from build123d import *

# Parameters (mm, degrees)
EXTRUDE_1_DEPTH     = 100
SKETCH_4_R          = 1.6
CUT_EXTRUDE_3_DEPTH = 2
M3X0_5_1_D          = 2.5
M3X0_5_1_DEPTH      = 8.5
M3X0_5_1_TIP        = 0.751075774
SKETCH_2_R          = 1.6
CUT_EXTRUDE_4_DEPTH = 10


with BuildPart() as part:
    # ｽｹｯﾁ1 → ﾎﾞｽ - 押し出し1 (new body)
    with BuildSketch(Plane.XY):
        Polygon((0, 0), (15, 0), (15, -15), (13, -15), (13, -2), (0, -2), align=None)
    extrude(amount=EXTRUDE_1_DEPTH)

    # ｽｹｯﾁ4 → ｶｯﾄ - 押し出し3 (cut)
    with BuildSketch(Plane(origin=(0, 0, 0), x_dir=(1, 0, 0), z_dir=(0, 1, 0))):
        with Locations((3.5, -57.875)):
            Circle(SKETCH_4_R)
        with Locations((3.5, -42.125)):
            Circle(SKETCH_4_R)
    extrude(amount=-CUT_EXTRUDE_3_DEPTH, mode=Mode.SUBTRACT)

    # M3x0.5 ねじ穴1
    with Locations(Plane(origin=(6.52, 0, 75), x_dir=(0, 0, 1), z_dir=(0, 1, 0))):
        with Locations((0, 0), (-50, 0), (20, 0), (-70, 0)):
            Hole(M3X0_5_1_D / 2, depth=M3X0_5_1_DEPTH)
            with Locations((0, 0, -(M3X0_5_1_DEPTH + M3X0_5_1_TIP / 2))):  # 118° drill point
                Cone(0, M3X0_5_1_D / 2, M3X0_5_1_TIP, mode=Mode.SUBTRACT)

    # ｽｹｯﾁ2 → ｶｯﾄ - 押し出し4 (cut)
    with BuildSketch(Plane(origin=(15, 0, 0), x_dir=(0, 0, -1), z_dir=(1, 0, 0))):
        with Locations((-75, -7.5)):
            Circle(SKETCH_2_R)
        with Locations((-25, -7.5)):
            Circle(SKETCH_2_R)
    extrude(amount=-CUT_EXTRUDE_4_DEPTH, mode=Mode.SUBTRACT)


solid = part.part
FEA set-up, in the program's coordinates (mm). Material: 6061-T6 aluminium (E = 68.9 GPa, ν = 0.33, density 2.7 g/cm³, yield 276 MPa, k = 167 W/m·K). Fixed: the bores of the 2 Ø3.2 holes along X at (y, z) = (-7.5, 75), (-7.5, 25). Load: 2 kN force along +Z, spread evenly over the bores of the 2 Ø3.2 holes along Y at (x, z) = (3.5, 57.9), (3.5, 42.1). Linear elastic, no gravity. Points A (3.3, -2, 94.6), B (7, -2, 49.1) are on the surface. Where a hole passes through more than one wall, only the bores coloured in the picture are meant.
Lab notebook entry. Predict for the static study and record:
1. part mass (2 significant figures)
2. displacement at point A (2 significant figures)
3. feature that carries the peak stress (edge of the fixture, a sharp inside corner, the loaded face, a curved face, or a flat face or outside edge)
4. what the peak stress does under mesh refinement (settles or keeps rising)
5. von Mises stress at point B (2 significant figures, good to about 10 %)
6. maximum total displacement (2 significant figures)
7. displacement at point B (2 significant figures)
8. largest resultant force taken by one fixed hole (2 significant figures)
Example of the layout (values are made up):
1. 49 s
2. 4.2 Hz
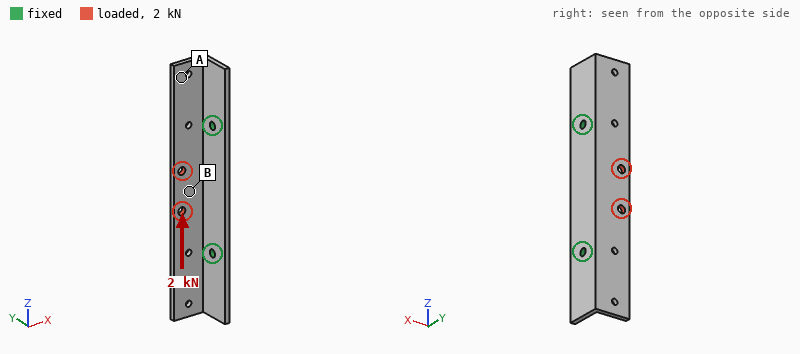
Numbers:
1. 15 g
2. 0.093 mm
3. edge of the fixture
4. keeps rising
5. 57 MPa
6. 0.12 mm
7. 0.026 mm
8. 1.1 kN
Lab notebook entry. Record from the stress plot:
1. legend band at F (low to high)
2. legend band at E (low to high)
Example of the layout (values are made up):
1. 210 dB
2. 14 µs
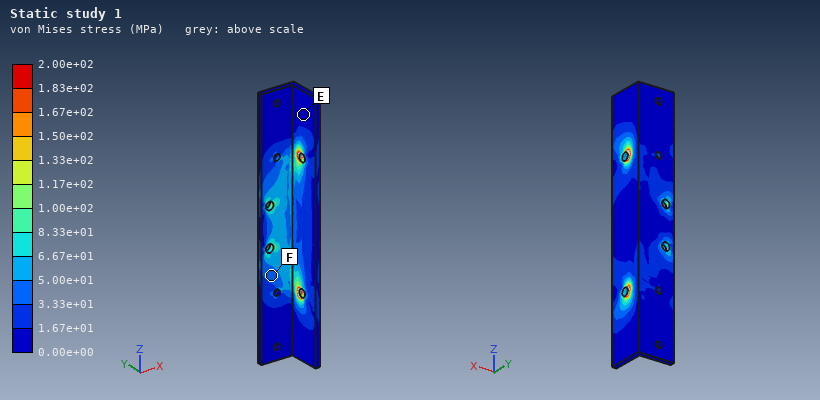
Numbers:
1. 3.33e+01 to 5.00e+01 MPa
2. 0.00e+00 to 1.67e+01 MPa
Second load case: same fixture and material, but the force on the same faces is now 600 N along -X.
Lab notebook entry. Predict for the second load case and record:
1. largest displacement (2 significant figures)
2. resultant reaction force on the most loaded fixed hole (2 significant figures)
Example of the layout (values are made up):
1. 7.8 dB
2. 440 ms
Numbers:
1. 0.11 mm
2. 380 N
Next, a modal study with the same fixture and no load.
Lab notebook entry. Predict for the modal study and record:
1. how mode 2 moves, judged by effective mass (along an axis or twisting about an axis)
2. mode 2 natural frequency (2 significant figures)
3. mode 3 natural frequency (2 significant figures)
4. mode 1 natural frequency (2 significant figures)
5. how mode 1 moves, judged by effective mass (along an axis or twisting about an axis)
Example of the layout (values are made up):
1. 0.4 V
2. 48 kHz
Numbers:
1. twisting about X
2. 4000 Hz
3. 5100 Hz
4. 3600 Hz
5. along Y
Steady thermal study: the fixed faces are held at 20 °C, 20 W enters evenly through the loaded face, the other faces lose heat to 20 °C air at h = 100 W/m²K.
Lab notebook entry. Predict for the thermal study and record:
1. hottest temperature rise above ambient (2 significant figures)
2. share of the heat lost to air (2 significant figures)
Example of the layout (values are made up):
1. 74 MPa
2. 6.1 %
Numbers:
1. 35 K
2. 29 %
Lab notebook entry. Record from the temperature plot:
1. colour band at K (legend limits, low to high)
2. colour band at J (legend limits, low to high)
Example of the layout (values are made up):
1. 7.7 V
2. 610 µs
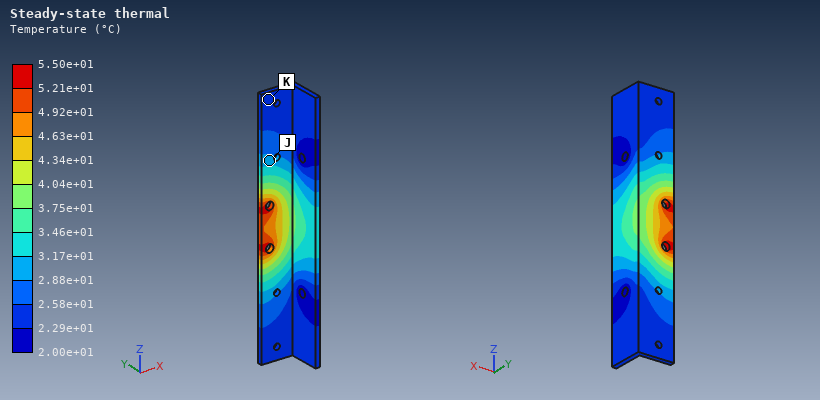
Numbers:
1. 2.29e+01 to 2.58e+01 °C
2. 2.88e+01 to 3.17e+01 °C
